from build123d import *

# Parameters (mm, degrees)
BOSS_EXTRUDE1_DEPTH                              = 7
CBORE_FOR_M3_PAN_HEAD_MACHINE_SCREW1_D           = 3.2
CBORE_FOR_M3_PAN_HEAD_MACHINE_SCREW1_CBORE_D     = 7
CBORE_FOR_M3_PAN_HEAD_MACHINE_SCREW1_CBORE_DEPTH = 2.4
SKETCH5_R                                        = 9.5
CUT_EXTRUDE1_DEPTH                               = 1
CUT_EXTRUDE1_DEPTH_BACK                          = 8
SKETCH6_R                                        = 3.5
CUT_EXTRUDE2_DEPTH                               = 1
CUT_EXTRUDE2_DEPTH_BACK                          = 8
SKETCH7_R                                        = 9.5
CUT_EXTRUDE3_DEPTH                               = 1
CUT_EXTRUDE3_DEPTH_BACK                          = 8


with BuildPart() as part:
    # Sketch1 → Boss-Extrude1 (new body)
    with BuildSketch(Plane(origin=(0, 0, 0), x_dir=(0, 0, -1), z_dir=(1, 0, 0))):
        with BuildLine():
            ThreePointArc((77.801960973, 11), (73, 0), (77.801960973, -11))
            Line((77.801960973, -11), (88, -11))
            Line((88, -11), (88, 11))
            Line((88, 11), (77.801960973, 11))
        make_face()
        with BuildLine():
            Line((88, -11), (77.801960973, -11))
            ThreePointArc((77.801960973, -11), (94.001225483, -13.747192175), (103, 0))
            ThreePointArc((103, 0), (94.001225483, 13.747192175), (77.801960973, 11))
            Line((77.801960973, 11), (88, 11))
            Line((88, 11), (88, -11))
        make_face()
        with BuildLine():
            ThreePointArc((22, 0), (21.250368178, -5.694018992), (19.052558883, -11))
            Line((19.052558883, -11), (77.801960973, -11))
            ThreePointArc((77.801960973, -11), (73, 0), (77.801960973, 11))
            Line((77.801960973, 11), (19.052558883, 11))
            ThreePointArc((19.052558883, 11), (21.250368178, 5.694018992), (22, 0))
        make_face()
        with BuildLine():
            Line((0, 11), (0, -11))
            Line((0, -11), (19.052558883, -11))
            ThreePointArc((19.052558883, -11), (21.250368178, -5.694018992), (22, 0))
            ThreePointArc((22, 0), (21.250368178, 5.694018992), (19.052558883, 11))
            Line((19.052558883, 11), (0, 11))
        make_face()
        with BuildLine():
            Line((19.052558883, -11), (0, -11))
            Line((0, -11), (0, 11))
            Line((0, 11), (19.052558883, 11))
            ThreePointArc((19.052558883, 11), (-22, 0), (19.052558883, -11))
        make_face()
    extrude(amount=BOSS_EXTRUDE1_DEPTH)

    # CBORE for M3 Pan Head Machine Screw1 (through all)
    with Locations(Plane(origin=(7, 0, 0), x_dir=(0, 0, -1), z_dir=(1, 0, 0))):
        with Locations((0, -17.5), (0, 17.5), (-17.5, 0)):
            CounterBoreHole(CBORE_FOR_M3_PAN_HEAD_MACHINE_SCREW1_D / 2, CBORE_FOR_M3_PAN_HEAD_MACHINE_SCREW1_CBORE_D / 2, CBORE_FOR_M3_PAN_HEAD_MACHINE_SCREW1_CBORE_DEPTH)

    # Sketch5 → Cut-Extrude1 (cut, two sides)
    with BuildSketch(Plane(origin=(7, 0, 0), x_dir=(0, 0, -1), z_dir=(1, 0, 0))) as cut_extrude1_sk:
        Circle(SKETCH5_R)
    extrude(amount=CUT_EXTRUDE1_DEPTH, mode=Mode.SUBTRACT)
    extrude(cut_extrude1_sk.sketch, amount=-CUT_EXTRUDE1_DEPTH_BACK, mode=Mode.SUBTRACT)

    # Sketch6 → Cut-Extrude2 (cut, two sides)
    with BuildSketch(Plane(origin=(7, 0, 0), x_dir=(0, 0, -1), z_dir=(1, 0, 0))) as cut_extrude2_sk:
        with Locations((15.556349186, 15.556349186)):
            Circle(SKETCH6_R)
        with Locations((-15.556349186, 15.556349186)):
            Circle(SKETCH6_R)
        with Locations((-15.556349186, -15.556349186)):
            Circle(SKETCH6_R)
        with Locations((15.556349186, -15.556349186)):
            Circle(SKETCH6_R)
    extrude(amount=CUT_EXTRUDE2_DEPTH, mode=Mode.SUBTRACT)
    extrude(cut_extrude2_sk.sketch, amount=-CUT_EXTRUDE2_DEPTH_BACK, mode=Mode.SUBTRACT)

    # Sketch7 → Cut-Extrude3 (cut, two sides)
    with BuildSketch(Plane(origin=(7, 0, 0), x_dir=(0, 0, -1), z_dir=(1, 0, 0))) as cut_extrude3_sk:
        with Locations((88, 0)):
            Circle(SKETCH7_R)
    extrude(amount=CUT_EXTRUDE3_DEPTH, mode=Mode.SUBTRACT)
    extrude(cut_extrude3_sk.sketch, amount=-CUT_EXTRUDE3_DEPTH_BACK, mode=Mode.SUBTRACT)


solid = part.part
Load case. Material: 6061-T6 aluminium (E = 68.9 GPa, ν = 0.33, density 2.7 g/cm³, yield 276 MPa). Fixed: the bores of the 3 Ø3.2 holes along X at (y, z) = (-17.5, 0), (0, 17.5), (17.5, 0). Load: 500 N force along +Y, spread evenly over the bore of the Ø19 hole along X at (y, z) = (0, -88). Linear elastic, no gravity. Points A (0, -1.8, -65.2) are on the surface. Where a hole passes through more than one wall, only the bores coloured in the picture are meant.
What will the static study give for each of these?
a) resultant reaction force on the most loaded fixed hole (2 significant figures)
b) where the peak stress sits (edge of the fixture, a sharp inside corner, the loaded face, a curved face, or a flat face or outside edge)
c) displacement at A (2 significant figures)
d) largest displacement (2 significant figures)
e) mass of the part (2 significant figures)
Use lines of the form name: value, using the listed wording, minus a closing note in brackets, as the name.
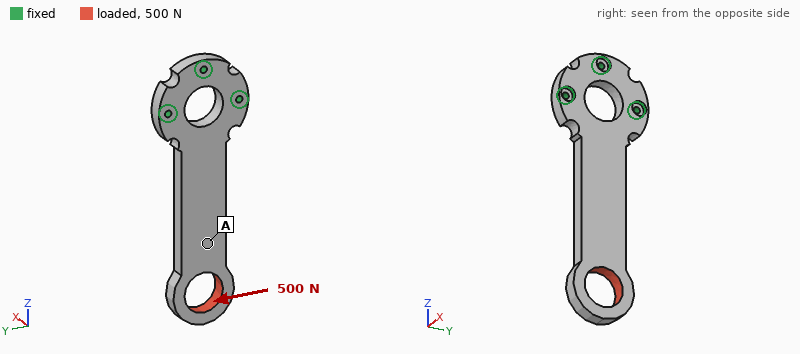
resultant reaction force on the most loaded fixed hole: 1.3 kN
where the peak stress sits: a curved face
displacement at A: 0.14 mm
largest displacement: 0.32 mm
mass of the part: 51 g
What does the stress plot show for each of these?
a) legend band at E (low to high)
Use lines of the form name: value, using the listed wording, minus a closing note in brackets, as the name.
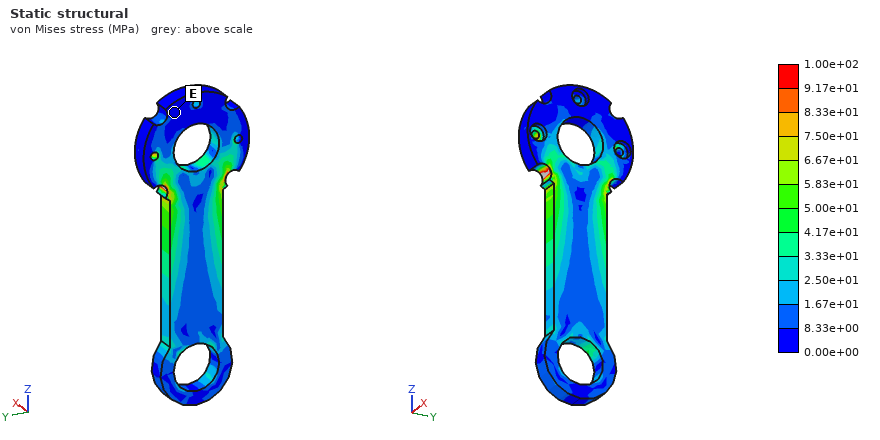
legend band at E: 0.00e+00 to 8.33e+00 MPa
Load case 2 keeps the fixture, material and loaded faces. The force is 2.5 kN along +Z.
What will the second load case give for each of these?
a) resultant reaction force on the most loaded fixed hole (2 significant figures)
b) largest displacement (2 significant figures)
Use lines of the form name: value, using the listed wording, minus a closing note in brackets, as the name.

resultant reaction force on the most loaded fixed hole: 1.3 kN
largest displacement: 63 µm
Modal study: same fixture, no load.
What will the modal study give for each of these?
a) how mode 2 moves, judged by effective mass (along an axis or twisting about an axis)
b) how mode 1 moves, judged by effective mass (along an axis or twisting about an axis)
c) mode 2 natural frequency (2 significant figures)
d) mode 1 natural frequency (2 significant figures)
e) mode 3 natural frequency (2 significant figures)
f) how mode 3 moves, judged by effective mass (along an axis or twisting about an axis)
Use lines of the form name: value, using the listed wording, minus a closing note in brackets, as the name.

how mode 2 moves, judged by effective mass: along Y
how mode 1 moves, judged by effective mass: along X
mode 2 natural frequency: 2100 Hz
mode 1 natural frequency: 550 Hz
mode 3 natural frequency: 3100 Hz
how mode 3 moves, judged by effective mass: along X
